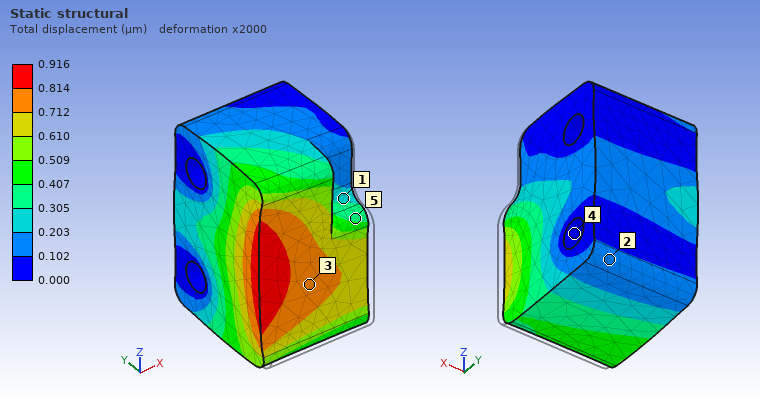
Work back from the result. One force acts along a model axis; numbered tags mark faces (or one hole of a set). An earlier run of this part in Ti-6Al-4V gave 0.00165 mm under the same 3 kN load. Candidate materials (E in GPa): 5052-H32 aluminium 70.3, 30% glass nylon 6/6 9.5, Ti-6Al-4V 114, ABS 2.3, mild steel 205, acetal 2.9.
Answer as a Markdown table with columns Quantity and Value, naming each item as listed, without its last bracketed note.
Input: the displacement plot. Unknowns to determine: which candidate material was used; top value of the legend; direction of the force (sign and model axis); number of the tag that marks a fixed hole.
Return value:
| Quantity | Value |
|---|---|
| which candidate material was used | mild steel |
| top value of the legend | 0.916 µm |
| direction of the force | +Y |
| number of the tag that marks a fixed hole | 4 |
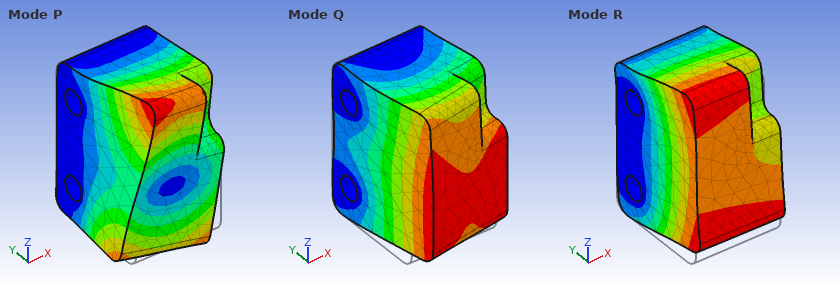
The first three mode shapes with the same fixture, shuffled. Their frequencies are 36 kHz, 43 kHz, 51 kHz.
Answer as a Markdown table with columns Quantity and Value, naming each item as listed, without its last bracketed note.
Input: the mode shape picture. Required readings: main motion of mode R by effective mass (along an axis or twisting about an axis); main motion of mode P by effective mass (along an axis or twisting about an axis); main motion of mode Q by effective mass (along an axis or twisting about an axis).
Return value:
| Quantity | Value |
|---|---|
| main motion of mode R by effective mass | along Z |
| main motion of mode P by effective mass | twisting about Y |
| main motion of mode Q by effective mass | along X |
